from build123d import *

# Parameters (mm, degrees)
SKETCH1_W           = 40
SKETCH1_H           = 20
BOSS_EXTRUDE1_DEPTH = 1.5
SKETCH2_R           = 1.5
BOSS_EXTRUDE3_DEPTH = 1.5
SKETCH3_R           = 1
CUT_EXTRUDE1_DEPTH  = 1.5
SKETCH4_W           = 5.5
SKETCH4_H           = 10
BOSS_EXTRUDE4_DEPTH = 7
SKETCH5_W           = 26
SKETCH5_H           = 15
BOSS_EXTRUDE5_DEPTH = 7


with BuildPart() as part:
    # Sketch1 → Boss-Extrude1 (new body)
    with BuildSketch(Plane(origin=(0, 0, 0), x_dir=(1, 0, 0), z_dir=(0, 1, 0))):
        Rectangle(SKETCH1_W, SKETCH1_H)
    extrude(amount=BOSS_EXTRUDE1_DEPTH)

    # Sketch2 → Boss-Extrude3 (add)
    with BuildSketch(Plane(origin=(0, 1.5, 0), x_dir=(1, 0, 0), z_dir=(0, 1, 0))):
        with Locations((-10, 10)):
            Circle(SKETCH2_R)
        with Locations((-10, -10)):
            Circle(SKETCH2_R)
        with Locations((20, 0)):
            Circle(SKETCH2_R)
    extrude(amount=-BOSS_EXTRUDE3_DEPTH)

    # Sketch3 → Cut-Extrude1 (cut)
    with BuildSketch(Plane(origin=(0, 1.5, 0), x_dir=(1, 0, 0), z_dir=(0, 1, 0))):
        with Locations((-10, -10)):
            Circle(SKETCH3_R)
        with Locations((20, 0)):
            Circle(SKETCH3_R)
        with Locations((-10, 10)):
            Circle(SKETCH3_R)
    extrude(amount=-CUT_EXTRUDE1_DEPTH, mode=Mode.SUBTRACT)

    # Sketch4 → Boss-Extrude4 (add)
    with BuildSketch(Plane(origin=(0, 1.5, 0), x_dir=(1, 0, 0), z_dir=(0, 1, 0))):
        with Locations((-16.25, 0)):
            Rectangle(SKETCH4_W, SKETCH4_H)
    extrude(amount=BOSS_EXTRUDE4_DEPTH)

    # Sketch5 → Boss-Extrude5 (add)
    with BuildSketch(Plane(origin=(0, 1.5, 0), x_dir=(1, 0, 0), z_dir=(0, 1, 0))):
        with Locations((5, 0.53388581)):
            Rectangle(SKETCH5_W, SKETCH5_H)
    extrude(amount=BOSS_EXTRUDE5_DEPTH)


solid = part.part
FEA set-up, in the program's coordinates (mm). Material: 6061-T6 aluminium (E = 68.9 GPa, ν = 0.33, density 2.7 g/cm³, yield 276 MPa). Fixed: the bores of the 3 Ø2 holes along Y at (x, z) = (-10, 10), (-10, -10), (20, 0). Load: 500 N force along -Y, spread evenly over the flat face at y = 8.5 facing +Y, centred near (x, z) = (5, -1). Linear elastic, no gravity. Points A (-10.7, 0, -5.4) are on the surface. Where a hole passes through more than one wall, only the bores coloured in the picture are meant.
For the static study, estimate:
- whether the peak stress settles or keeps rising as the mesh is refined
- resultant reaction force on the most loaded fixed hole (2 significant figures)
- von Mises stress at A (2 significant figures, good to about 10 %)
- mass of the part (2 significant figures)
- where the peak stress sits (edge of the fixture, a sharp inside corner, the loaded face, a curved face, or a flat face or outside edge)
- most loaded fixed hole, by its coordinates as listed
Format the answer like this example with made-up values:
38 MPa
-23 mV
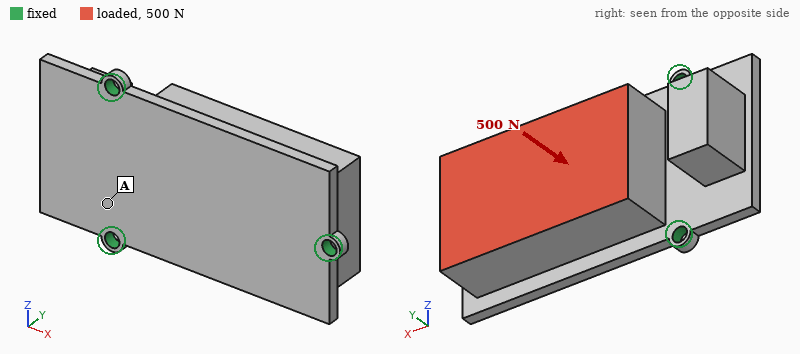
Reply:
keeps rising
290 N
18 MPa
12 g
edge of the fixture
(20, 0)
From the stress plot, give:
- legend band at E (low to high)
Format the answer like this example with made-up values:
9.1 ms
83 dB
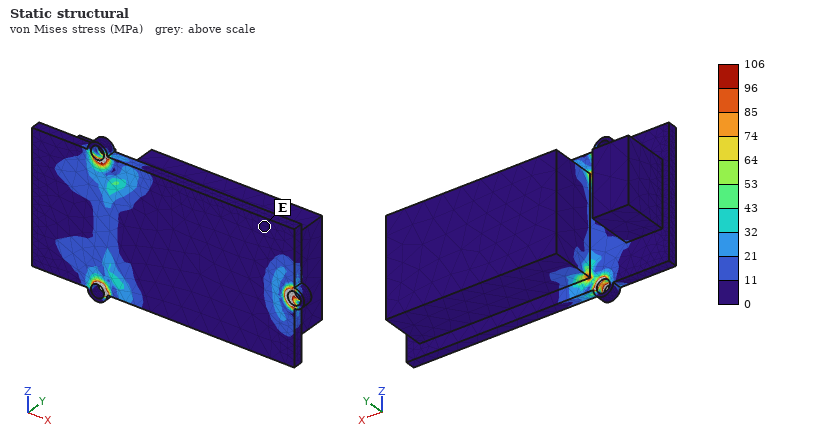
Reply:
0 to 11 MPa
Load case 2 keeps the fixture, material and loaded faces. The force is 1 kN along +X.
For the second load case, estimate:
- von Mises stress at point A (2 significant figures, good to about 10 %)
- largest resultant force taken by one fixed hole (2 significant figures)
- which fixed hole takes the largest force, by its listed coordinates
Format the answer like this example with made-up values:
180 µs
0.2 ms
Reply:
22 MPa
550 N
(20, 0)
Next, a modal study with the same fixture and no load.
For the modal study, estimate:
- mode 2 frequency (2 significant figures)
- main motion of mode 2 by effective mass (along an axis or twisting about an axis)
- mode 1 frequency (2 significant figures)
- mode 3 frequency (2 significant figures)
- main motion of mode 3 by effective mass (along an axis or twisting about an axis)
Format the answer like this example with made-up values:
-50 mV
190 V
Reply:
9900 Hz
along Z
5400 Hz
12 kHz
along Y
